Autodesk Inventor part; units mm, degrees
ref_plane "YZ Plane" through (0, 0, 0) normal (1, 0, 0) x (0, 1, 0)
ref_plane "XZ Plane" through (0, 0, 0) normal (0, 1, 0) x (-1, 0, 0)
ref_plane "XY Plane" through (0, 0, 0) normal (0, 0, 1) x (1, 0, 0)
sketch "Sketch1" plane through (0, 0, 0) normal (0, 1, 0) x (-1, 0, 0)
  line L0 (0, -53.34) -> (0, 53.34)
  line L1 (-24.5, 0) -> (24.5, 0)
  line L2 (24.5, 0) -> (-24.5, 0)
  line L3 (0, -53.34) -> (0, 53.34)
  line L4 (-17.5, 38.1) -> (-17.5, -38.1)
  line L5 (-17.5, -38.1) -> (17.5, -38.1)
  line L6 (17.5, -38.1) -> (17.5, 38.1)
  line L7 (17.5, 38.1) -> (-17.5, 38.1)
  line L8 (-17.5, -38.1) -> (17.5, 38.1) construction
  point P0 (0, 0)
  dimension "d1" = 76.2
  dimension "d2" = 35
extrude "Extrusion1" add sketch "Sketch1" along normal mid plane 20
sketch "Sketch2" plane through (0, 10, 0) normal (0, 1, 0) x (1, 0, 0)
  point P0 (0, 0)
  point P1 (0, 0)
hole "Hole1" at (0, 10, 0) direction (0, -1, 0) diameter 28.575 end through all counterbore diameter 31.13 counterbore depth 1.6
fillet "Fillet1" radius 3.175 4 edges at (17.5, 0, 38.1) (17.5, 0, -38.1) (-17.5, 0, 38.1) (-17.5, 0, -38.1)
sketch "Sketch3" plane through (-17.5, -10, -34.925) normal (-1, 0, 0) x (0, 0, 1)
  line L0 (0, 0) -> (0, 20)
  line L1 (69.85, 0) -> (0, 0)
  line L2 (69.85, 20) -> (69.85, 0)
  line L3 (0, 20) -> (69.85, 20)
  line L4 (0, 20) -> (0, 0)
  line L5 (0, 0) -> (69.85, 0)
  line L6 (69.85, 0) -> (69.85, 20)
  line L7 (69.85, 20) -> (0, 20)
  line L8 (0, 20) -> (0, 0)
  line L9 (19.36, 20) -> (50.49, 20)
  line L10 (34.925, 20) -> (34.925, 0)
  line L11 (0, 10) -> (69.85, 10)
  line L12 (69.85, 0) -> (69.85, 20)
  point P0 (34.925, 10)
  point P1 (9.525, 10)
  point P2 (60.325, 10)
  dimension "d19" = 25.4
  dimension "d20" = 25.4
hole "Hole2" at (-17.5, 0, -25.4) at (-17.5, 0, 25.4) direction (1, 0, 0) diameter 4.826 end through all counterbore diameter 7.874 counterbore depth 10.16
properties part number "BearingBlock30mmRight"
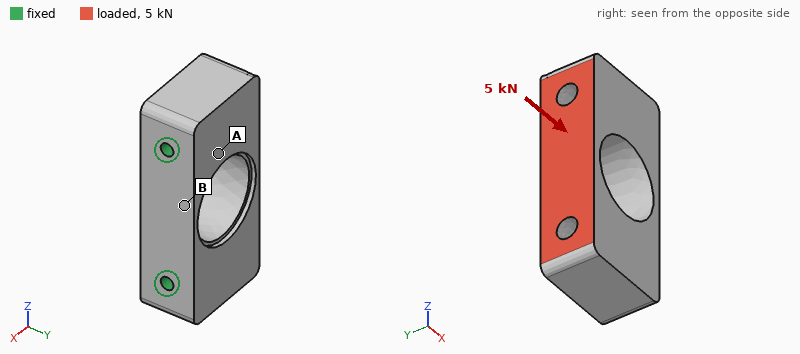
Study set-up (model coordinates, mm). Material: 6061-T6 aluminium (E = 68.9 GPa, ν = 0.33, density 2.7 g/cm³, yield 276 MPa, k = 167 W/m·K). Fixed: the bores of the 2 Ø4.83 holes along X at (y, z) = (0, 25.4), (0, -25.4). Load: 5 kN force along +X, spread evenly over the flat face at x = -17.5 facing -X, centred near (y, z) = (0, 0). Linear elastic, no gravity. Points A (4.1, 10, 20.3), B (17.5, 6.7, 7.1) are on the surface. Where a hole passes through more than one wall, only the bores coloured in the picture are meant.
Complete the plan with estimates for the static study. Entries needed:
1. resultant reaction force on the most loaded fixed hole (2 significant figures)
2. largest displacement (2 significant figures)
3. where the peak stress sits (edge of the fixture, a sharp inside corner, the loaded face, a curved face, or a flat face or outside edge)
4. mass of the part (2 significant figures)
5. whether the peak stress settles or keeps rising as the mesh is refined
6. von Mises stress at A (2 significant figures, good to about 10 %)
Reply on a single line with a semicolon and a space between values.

2.6 kN; 12 µm; edge of the fixture; 100 g; keeps rising; 5.7 MPa
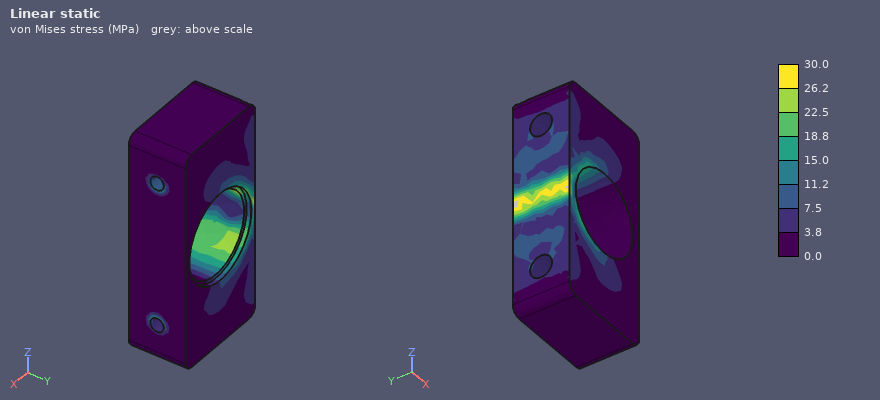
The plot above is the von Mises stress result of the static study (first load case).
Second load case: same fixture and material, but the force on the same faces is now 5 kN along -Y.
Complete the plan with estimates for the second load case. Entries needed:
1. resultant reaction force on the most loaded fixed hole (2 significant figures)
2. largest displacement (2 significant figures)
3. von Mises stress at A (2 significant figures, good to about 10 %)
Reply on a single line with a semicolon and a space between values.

2.5 kN; 32 µm; 17 MPa
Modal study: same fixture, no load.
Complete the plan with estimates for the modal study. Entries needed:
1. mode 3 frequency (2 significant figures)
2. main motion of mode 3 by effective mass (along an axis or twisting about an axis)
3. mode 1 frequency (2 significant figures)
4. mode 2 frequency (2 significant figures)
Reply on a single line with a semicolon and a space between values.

23 kHz; along Z; 16 kHz; 21 kHz
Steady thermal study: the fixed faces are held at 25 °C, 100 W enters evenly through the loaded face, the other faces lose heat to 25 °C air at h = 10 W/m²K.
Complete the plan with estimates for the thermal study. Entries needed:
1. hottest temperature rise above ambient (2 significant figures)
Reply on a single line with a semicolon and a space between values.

22 K
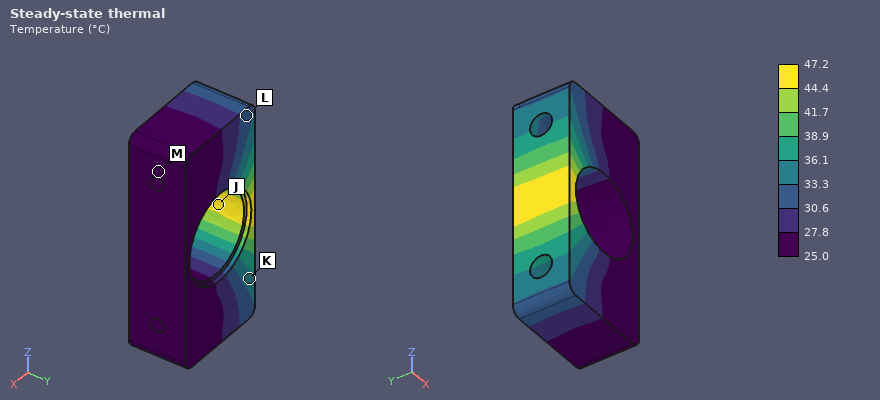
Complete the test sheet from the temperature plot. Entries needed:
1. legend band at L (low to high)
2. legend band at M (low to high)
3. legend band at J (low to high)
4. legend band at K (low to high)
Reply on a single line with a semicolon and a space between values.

30.6 to 33.3 °C; 25.0 to 27.8 °C; 44.4 to 47.2 °C; 33.3 to 36.1 °C
